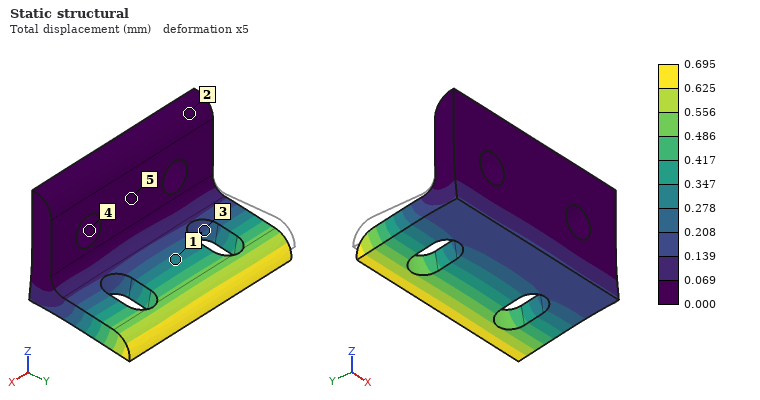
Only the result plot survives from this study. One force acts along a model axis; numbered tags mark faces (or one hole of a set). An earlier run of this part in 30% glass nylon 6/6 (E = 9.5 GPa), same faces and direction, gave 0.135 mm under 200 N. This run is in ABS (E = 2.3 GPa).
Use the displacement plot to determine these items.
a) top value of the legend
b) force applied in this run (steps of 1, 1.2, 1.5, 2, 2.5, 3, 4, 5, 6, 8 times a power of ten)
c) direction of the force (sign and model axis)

0.695 mm
250 N
-Z
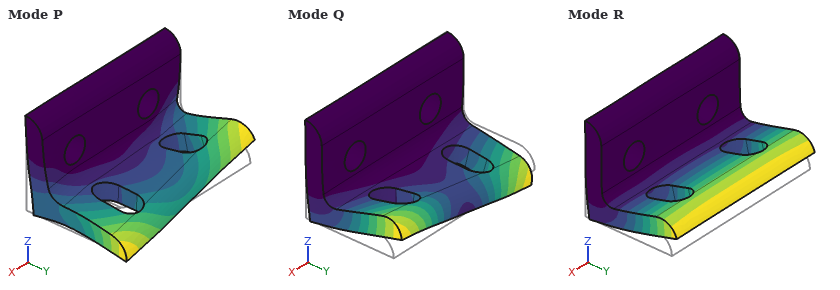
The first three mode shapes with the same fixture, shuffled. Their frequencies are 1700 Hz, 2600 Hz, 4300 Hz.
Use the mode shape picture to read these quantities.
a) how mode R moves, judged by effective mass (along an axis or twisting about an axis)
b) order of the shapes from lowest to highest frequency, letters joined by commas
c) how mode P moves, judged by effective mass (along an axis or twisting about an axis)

along Z
R, Q, P
along X
